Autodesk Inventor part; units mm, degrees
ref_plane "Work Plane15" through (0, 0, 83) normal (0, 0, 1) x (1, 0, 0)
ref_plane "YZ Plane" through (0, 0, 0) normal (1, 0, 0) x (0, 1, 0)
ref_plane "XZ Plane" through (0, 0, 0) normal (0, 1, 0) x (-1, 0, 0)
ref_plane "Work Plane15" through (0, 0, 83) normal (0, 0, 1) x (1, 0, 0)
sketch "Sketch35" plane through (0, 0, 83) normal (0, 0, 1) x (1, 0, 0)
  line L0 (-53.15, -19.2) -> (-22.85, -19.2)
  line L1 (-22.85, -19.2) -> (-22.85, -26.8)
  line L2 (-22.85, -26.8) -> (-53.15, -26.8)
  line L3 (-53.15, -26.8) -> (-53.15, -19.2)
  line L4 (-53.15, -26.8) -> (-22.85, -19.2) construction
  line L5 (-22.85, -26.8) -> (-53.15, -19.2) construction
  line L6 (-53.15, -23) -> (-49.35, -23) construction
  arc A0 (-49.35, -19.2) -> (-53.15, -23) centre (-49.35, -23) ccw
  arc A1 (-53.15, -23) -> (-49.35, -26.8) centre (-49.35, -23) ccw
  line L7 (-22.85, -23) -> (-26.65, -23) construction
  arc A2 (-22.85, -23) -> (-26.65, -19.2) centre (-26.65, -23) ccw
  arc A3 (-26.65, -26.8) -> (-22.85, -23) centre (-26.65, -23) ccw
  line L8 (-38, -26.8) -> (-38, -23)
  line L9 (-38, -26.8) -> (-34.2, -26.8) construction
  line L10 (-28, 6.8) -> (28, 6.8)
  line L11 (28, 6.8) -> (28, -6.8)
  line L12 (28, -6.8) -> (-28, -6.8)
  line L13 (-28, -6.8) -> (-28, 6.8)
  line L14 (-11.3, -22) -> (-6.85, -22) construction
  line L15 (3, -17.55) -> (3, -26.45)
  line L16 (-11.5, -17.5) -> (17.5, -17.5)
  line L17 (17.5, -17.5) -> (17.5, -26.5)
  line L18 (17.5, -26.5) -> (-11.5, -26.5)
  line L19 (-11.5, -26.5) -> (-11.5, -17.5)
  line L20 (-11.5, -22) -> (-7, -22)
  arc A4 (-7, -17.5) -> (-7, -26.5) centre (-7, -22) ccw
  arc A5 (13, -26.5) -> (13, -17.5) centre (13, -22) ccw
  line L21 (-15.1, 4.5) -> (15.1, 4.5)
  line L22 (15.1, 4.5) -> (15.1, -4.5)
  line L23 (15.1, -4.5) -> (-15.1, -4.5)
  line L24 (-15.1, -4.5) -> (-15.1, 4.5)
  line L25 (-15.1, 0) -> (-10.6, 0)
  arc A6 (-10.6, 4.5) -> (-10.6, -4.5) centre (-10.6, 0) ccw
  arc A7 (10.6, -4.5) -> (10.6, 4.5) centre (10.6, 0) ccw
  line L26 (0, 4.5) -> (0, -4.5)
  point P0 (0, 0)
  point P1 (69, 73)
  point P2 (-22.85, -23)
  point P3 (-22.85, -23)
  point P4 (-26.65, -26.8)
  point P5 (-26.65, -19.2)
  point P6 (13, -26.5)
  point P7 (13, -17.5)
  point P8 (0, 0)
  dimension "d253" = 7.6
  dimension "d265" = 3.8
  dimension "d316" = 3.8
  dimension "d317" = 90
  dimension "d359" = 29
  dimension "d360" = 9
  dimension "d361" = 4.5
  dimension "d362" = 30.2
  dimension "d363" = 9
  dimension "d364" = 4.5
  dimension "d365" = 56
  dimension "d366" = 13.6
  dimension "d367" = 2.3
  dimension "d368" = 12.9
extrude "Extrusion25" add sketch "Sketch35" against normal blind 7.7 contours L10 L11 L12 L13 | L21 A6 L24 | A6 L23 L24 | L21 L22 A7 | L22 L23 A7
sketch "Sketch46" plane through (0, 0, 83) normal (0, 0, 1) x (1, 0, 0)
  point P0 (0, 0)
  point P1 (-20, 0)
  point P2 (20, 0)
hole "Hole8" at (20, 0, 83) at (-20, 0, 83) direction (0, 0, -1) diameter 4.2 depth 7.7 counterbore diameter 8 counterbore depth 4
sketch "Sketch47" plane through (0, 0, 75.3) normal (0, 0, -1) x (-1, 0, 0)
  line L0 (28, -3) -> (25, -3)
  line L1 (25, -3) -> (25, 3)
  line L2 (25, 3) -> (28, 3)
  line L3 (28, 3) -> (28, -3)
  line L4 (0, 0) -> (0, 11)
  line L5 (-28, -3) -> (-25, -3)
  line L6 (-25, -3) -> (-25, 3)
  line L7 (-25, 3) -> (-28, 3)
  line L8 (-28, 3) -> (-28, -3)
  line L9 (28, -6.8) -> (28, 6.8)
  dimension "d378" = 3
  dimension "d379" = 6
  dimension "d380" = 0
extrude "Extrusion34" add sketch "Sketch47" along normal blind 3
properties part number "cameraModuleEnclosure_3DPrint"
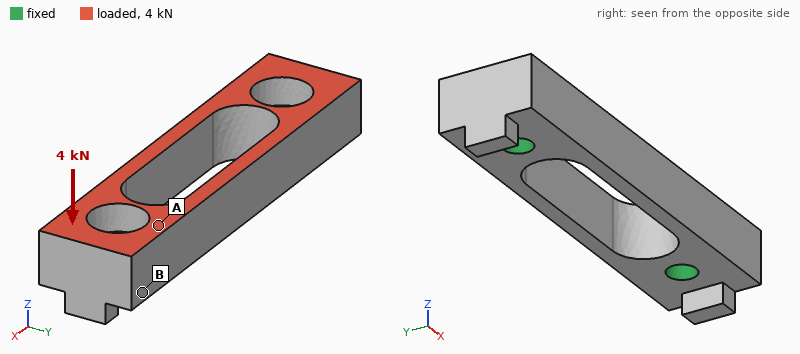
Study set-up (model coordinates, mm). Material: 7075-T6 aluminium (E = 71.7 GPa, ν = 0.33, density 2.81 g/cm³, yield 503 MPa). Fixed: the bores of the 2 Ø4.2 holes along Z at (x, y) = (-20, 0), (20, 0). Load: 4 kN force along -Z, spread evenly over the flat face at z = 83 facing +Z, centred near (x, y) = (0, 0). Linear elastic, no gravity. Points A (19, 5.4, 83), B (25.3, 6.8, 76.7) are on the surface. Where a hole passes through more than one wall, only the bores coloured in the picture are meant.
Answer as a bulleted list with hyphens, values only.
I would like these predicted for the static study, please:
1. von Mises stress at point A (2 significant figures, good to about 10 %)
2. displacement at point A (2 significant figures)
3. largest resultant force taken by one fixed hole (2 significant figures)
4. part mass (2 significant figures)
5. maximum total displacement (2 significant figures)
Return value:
- 50 MPa
- 8.4 µm
- 2.0 kN
- 9.9 g
- 38 µm
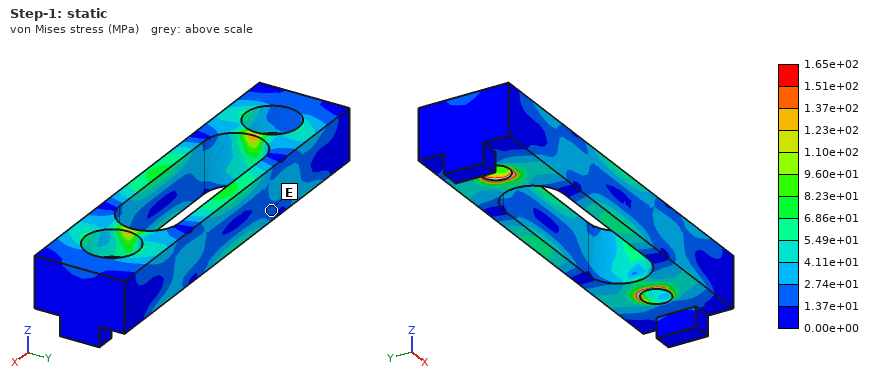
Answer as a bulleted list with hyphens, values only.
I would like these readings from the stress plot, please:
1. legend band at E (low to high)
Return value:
- 1.37e+01 to 2.74e+01 MPa
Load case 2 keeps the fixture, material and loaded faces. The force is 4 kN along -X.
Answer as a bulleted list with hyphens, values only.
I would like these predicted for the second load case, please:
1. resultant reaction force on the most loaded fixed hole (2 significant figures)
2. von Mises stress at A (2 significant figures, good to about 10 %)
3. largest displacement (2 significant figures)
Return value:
- 2.0 kN
- 29 MPa
- 22 µm
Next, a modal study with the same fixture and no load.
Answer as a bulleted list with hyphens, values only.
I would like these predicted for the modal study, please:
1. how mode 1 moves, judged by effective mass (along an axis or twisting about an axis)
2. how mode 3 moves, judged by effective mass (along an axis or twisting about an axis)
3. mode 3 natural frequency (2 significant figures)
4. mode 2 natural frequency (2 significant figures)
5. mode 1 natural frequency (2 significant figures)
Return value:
- along Y
- along Z
- 19 kHz
- 14 kHz
- 14 kHz
